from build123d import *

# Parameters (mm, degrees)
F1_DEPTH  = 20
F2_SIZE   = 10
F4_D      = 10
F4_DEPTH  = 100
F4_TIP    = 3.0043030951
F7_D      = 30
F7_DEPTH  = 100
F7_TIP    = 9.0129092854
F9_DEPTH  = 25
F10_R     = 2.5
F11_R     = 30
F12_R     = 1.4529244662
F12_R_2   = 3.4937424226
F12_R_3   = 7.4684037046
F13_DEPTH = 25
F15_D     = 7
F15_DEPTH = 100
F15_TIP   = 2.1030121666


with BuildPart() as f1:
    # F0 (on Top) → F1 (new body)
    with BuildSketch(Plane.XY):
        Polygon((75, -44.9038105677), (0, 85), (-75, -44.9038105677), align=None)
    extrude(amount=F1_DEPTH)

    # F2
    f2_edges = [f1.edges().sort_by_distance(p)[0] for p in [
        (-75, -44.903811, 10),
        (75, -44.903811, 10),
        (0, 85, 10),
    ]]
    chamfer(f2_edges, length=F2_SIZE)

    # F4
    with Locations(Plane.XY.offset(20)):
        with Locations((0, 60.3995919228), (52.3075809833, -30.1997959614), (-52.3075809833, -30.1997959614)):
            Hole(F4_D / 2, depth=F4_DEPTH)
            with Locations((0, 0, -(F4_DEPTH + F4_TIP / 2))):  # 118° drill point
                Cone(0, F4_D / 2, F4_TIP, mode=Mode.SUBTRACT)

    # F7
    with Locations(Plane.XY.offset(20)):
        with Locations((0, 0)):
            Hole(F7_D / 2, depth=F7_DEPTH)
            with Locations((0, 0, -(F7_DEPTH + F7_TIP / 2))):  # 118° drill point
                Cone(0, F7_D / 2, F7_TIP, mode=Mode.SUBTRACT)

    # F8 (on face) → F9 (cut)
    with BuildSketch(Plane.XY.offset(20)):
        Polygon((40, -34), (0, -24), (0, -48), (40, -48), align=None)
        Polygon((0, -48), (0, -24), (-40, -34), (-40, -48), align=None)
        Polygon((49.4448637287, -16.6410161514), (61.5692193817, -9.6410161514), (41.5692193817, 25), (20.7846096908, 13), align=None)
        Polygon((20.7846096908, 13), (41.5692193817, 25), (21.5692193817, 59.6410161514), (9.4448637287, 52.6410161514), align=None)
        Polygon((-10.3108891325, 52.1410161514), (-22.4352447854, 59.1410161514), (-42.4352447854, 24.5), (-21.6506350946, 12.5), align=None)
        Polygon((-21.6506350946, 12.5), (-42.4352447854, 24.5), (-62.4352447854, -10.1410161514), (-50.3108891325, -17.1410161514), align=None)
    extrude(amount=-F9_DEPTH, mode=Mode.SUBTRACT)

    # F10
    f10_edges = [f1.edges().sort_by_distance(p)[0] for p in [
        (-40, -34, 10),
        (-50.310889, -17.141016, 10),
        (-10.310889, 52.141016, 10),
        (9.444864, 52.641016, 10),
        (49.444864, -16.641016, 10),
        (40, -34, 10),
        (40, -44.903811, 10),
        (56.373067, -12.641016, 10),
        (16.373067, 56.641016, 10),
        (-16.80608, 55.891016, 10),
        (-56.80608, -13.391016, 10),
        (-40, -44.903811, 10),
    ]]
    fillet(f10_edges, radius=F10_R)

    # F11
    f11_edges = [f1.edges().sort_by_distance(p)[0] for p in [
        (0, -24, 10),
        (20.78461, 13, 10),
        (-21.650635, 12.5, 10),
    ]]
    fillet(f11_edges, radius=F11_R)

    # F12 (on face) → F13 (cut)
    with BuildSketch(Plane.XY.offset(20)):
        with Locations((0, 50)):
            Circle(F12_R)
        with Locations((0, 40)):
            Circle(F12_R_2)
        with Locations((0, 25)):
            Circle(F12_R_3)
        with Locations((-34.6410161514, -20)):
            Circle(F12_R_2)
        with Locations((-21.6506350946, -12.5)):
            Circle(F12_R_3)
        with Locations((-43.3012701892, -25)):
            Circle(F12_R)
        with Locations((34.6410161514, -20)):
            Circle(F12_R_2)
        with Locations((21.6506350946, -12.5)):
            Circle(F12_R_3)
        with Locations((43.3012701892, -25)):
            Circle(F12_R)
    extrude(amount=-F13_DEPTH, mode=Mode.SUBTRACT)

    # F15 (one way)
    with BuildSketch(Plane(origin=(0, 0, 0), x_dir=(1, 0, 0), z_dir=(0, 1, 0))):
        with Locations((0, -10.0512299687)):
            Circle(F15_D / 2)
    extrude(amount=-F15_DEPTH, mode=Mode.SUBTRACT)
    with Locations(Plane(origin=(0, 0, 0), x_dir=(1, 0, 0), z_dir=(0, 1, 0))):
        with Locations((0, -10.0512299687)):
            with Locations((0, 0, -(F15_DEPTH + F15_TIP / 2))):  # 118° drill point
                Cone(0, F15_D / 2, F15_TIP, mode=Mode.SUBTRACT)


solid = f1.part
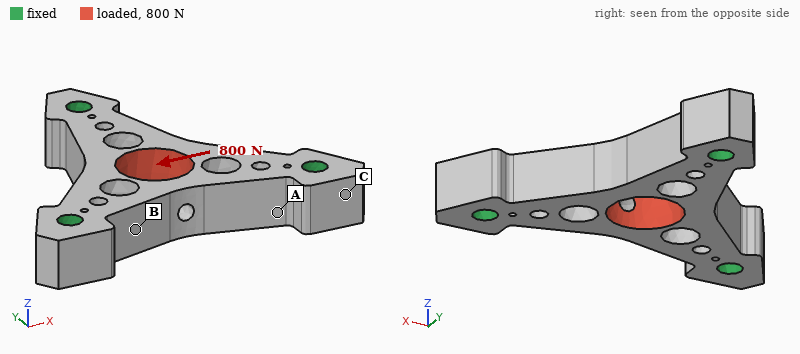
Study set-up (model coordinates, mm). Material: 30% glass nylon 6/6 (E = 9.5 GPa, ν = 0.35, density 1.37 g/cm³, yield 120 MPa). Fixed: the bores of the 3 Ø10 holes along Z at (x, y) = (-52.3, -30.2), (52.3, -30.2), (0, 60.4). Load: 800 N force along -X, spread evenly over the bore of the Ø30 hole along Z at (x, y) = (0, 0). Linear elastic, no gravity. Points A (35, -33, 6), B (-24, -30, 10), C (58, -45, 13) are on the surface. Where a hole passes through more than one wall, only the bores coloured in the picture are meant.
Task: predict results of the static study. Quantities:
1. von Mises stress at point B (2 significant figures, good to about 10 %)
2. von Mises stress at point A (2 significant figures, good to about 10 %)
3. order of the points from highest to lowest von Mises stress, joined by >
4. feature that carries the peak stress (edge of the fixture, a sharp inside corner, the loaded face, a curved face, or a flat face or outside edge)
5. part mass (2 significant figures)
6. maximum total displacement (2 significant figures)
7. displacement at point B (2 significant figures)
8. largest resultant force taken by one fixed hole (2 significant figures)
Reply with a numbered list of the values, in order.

1. 1.3 MPa
2. 0.78 MPa
3. B > A > C
4. a curved face
5. 130 g
6. 13 µm
7. 3.0 µm
8. 400 N
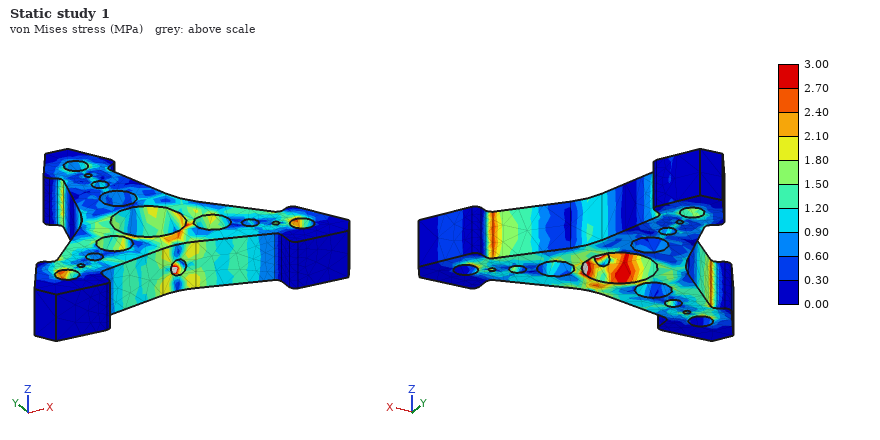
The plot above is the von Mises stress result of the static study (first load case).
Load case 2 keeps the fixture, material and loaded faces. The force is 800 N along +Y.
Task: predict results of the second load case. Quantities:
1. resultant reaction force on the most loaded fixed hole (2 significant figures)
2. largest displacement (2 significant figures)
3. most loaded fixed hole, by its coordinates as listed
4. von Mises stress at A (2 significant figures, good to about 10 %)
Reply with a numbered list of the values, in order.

1. 470 N
2. 14 µm
3. (0, 60.4)
4. 1.5 MPa
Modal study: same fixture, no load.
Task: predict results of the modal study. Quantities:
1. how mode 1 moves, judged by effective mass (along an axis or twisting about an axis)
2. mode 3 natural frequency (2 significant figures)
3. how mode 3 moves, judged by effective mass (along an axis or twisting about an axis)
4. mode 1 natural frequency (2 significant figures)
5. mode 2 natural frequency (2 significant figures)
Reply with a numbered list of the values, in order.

1. along Z
2. 5800 Hz
3. along Y
4. 3900 Hz
5. 5600 Hz
